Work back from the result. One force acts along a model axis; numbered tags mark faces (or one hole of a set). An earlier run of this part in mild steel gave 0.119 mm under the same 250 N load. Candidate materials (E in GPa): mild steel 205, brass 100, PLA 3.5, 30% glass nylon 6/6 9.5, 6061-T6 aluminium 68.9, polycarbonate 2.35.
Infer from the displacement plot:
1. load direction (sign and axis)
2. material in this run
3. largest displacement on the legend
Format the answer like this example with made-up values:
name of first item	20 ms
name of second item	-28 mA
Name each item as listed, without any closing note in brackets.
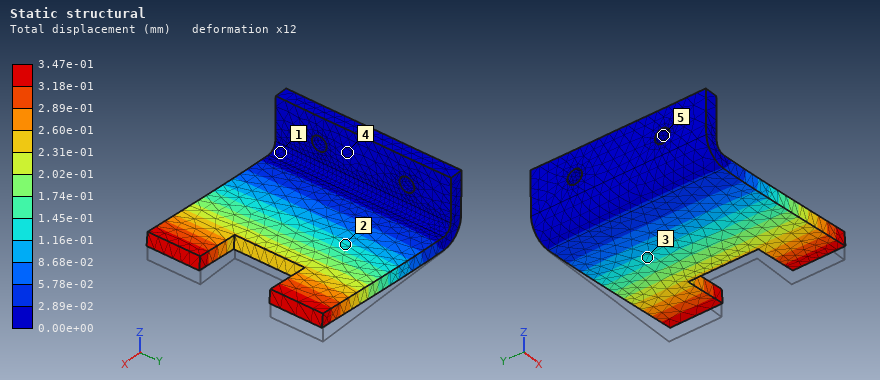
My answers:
load direction	+Z
material in this run	6061-T6 aluminium
largest displacement on the legend	3.47e-01 mm
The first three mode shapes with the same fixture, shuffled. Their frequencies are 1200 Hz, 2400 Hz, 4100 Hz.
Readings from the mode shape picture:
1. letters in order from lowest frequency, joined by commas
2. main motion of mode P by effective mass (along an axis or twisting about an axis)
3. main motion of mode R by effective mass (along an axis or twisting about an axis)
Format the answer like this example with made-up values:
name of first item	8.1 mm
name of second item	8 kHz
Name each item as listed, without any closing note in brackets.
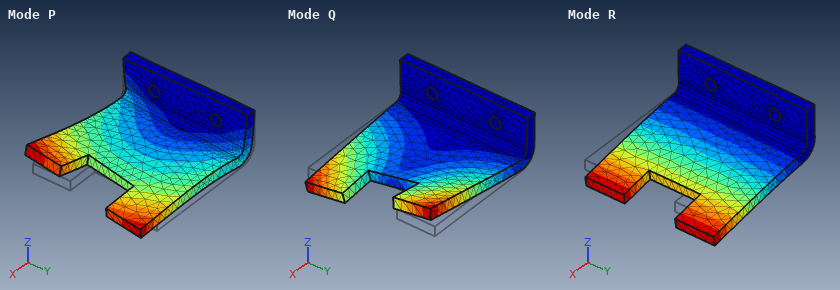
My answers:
letters in order from lowest frequency, joined by commas	R, Q, P
main motion of mode P by effective mass	along Y
main motion of mode R by effective mass	along Z
